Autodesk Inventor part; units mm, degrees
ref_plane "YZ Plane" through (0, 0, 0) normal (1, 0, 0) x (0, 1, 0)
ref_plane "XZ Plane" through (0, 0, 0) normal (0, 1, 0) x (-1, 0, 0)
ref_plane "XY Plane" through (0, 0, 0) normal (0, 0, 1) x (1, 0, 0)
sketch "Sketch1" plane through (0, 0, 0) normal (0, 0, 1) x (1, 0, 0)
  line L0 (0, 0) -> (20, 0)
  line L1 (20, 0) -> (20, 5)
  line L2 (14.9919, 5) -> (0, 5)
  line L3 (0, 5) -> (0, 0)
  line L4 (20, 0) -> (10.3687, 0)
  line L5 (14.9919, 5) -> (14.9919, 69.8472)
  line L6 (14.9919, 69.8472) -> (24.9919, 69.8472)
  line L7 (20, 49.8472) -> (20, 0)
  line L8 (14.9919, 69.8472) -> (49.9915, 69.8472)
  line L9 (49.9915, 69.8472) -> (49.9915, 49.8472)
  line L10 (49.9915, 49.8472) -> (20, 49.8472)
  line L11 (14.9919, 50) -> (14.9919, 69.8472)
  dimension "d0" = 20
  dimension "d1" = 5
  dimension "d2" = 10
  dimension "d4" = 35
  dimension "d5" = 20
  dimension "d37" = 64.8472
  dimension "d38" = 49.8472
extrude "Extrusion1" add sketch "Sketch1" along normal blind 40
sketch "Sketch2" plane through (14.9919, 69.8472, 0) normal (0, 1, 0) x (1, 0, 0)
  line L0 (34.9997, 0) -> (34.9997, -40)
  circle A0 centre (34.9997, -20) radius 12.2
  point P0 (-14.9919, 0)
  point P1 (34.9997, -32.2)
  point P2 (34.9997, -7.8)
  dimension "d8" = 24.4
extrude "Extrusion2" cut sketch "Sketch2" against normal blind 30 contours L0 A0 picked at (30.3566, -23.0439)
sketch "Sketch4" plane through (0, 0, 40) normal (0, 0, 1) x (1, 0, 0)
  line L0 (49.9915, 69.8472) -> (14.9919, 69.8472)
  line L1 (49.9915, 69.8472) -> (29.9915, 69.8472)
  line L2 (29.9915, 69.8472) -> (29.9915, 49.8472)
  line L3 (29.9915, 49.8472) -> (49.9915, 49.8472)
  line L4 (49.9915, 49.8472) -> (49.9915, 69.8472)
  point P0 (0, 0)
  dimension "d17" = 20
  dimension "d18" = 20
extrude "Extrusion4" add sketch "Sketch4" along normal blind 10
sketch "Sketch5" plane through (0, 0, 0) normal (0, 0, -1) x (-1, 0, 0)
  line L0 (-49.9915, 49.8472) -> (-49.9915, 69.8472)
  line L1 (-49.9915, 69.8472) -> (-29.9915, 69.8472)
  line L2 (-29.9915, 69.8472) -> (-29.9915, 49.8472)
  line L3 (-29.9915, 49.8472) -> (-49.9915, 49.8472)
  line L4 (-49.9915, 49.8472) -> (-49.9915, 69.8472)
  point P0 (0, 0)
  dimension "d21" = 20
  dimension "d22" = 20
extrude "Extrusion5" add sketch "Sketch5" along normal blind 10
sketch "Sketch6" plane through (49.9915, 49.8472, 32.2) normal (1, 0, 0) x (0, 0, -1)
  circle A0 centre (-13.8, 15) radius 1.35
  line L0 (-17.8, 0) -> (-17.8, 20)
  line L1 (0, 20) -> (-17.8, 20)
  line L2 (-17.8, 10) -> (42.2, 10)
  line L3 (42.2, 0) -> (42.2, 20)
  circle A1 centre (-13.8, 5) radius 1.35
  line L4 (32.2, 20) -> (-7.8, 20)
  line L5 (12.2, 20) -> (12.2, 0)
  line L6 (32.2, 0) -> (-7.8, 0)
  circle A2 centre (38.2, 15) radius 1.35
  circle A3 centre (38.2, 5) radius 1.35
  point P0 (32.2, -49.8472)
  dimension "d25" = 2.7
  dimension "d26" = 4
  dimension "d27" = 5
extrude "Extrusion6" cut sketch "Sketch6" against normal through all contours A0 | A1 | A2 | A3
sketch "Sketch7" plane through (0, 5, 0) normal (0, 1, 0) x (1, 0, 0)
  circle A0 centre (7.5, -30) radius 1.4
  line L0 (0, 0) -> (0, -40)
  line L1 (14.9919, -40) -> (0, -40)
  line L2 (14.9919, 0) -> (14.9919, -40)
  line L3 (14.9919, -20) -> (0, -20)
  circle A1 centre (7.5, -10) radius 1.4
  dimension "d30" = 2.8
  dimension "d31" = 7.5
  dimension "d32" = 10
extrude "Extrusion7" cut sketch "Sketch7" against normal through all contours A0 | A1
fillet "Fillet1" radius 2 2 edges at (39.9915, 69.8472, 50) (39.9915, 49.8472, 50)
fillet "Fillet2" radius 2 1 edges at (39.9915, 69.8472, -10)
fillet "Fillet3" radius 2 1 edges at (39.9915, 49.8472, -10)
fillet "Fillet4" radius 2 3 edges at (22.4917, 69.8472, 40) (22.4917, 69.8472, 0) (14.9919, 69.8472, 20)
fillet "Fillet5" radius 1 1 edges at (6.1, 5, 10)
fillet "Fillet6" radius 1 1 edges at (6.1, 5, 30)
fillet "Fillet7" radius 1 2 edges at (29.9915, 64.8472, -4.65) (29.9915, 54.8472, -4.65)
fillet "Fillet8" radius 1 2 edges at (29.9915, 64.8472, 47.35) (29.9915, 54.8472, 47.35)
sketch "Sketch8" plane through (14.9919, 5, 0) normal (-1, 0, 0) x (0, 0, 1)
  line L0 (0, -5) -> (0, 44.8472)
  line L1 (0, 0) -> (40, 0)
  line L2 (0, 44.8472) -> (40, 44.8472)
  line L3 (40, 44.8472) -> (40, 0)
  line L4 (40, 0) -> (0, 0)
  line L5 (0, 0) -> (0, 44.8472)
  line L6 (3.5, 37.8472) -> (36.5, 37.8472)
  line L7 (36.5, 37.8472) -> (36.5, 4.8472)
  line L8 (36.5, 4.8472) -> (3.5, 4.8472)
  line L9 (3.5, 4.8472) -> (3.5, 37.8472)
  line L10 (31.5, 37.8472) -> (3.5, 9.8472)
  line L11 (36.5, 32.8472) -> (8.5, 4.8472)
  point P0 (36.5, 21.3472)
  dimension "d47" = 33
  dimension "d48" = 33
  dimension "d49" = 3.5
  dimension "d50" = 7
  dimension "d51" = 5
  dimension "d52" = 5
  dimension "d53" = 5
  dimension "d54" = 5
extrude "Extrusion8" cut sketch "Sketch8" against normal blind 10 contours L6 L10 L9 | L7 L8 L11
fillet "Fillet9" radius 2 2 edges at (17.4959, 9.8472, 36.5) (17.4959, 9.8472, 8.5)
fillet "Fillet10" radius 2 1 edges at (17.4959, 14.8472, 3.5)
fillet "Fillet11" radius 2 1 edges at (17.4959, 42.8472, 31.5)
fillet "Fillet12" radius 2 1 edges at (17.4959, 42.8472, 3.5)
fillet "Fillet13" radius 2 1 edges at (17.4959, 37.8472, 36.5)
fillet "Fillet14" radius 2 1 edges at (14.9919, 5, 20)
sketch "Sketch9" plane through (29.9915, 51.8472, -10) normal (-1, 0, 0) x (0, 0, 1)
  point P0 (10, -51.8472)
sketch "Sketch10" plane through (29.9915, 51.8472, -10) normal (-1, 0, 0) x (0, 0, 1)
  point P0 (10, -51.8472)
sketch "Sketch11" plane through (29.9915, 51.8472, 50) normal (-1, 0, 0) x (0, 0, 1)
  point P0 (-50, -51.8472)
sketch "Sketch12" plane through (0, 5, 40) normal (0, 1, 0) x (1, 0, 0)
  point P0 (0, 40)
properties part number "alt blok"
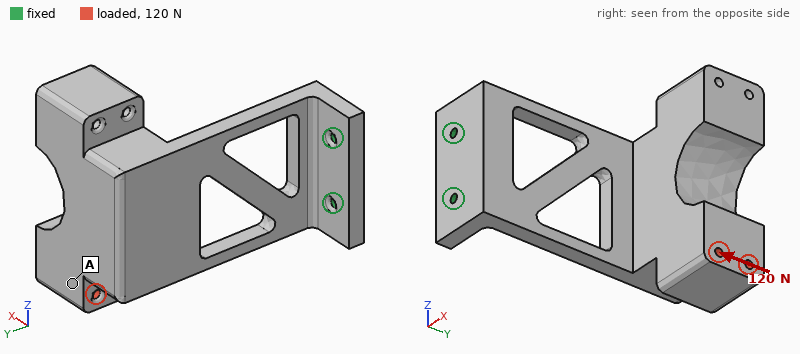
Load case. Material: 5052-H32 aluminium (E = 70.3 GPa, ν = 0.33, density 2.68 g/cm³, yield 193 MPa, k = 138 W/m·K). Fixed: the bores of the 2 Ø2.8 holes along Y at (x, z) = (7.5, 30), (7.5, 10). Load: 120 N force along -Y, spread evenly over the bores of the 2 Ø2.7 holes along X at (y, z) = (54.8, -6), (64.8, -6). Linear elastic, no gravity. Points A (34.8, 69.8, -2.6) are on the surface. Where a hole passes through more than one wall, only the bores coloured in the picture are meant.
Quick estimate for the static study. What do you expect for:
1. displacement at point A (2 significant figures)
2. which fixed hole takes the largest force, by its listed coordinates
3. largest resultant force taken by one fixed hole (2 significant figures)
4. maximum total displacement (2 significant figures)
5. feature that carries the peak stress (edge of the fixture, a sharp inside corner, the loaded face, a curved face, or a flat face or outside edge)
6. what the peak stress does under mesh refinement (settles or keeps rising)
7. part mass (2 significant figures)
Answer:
0.69 mm
(7.5, 10)
180 N
0.80 mm
edge of the fixture
keeps rising
110 g
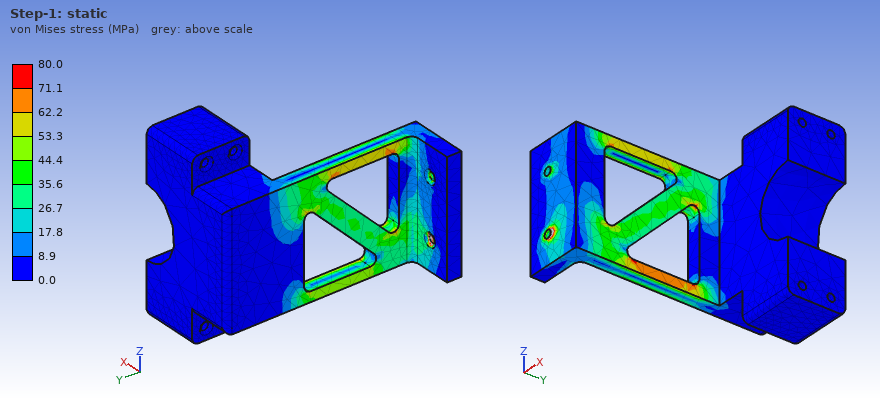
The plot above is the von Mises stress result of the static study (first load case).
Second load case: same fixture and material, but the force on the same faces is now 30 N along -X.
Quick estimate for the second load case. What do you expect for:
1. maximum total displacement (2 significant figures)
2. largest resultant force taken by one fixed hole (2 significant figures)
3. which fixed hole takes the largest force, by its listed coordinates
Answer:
0.35 mm
51 N
(7.5, 10)
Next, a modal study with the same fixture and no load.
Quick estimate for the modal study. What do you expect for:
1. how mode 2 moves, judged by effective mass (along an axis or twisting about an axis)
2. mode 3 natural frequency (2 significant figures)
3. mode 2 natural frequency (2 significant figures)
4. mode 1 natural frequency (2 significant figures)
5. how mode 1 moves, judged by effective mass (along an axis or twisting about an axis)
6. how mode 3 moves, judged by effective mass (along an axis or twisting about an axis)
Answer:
along Z
1000 Hz
500 Hz
190 Hz
along X
along Z
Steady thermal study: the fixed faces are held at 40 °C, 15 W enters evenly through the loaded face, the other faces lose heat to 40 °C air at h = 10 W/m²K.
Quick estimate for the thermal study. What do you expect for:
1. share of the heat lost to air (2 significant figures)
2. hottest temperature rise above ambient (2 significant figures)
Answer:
33 %
62 K
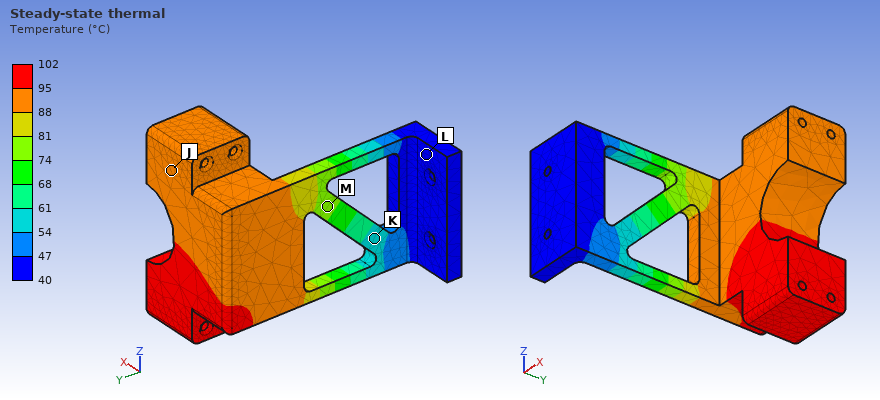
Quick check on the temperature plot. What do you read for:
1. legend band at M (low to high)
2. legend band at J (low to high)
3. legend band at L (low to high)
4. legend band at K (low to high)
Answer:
74 to 81 °C
88 to 95 °C
40 to 47 °C
54 to 61 °C
